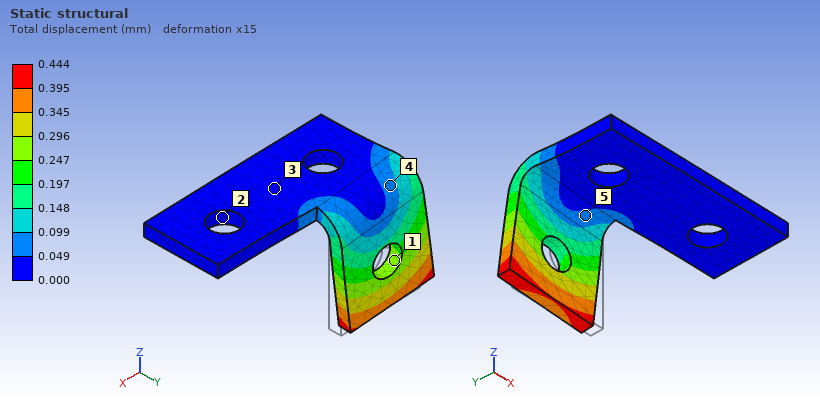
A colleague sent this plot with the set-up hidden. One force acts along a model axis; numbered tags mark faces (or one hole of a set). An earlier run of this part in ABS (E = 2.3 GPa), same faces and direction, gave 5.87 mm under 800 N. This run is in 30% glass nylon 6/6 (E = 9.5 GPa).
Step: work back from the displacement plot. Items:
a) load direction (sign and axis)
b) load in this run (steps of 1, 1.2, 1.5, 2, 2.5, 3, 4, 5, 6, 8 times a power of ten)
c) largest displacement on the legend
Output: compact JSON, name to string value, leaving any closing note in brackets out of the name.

{"load direction": "-X", "load in this run": "250 N", "largest displacement on the legend": "0.444 mm"}
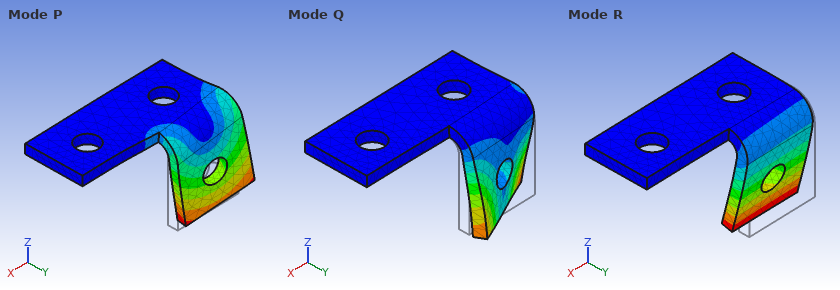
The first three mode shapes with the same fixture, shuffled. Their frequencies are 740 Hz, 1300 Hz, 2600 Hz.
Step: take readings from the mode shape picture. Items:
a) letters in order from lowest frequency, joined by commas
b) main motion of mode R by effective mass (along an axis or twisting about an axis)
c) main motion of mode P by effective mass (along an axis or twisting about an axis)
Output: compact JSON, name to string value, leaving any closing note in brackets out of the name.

{"letters in order from lowest frequency, joined by commas": "R, P, Q", "main motion of mode R by effective mass": "along Y", "main motion of mode P by effective mass": "along X"}
